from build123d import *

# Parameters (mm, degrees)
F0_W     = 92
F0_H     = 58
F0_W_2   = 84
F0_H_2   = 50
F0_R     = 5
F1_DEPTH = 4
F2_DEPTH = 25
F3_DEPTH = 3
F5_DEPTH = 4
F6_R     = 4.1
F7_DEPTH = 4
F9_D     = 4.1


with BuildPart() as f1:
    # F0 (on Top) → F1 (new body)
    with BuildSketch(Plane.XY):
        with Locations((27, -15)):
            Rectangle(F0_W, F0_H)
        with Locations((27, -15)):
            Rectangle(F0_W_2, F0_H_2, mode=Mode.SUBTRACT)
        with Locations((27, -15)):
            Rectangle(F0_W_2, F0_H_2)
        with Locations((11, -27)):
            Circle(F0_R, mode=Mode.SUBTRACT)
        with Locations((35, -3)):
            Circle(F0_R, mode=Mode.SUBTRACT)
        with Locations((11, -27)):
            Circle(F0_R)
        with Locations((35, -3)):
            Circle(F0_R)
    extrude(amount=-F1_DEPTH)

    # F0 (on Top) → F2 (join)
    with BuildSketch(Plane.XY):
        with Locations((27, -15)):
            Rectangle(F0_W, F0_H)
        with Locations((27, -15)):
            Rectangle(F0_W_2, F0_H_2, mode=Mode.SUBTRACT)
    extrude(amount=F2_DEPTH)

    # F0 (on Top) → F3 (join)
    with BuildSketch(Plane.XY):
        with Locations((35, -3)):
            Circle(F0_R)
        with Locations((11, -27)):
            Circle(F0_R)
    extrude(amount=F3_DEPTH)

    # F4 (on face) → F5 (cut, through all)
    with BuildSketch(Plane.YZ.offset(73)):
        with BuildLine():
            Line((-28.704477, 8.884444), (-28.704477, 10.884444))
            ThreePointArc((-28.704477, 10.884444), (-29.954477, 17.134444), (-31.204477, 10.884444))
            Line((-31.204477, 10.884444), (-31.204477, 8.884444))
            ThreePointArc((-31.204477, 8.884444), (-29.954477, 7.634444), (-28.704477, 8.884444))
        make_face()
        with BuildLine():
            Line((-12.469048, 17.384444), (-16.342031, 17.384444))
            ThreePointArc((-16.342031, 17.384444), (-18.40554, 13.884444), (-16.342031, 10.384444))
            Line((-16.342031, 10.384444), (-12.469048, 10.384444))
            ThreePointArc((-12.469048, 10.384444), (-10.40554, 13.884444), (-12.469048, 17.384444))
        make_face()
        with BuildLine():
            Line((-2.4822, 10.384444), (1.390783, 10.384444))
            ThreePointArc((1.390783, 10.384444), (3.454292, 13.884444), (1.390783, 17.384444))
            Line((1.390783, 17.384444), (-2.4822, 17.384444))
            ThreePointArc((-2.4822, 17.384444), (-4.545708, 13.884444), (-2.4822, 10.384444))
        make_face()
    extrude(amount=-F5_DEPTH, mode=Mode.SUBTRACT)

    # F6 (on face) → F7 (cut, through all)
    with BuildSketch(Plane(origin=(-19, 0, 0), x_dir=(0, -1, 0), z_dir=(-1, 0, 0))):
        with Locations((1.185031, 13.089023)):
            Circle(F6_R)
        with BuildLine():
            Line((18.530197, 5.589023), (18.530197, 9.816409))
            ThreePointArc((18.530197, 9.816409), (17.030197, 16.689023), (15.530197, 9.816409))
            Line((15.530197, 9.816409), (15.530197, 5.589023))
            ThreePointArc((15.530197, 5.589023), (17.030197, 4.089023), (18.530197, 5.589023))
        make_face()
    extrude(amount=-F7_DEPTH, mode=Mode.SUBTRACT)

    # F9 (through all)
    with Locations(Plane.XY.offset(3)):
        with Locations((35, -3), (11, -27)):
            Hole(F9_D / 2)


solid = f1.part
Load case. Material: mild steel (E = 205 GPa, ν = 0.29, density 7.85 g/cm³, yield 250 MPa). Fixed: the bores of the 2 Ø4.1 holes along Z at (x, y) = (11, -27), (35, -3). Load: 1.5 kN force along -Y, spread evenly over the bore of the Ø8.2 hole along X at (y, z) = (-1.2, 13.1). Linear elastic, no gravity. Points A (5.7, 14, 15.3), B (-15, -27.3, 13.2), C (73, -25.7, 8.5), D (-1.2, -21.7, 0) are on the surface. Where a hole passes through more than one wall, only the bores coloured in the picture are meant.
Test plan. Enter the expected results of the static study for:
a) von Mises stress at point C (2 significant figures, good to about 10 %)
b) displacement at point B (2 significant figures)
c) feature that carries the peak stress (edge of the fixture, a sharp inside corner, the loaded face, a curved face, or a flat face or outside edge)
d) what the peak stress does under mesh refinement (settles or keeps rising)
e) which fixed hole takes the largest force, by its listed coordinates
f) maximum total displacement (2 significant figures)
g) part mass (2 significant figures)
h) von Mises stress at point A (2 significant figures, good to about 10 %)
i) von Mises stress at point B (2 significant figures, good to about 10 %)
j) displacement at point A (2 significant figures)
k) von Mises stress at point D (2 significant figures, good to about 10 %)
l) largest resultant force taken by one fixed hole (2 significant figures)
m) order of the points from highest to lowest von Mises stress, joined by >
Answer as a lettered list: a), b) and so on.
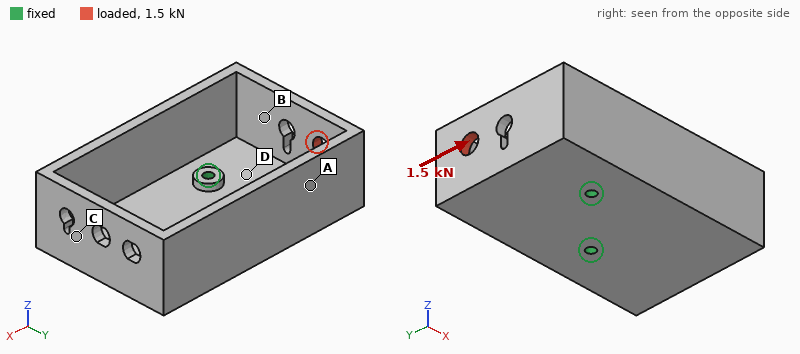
a) 16 MPa
b) 0.036 mm
c) edge of the fixture
d) keeps rising
e) (11, -27)
f) 0.11 mm
g) 390 g
h) 22 MPa
i) 31 MPa
j) 0.061 mm
k) 50 MPa
l) 2.3 kN
m) D > B > A > C
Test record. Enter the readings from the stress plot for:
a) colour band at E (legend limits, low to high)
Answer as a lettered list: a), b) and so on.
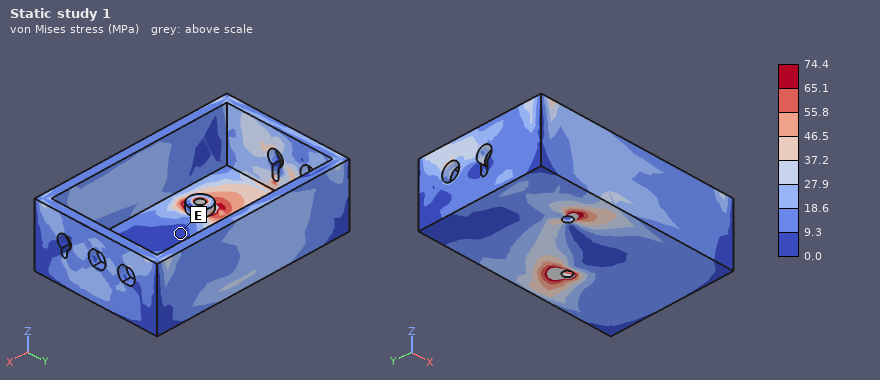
a) 0.0 to 9.3 MPa
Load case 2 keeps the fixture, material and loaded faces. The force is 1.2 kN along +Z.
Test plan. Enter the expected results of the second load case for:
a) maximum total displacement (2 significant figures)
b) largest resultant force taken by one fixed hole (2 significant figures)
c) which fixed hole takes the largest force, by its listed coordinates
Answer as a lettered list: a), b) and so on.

a) 0.22 mm
b) 1000 N
c) (11, -27)
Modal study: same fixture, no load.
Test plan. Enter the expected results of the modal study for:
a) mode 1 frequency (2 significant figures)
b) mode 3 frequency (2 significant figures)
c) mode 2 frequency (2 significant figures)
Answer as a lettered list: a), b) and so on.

a) 1100 Hz
b) 2600 Hz
c) 1800 Hz
